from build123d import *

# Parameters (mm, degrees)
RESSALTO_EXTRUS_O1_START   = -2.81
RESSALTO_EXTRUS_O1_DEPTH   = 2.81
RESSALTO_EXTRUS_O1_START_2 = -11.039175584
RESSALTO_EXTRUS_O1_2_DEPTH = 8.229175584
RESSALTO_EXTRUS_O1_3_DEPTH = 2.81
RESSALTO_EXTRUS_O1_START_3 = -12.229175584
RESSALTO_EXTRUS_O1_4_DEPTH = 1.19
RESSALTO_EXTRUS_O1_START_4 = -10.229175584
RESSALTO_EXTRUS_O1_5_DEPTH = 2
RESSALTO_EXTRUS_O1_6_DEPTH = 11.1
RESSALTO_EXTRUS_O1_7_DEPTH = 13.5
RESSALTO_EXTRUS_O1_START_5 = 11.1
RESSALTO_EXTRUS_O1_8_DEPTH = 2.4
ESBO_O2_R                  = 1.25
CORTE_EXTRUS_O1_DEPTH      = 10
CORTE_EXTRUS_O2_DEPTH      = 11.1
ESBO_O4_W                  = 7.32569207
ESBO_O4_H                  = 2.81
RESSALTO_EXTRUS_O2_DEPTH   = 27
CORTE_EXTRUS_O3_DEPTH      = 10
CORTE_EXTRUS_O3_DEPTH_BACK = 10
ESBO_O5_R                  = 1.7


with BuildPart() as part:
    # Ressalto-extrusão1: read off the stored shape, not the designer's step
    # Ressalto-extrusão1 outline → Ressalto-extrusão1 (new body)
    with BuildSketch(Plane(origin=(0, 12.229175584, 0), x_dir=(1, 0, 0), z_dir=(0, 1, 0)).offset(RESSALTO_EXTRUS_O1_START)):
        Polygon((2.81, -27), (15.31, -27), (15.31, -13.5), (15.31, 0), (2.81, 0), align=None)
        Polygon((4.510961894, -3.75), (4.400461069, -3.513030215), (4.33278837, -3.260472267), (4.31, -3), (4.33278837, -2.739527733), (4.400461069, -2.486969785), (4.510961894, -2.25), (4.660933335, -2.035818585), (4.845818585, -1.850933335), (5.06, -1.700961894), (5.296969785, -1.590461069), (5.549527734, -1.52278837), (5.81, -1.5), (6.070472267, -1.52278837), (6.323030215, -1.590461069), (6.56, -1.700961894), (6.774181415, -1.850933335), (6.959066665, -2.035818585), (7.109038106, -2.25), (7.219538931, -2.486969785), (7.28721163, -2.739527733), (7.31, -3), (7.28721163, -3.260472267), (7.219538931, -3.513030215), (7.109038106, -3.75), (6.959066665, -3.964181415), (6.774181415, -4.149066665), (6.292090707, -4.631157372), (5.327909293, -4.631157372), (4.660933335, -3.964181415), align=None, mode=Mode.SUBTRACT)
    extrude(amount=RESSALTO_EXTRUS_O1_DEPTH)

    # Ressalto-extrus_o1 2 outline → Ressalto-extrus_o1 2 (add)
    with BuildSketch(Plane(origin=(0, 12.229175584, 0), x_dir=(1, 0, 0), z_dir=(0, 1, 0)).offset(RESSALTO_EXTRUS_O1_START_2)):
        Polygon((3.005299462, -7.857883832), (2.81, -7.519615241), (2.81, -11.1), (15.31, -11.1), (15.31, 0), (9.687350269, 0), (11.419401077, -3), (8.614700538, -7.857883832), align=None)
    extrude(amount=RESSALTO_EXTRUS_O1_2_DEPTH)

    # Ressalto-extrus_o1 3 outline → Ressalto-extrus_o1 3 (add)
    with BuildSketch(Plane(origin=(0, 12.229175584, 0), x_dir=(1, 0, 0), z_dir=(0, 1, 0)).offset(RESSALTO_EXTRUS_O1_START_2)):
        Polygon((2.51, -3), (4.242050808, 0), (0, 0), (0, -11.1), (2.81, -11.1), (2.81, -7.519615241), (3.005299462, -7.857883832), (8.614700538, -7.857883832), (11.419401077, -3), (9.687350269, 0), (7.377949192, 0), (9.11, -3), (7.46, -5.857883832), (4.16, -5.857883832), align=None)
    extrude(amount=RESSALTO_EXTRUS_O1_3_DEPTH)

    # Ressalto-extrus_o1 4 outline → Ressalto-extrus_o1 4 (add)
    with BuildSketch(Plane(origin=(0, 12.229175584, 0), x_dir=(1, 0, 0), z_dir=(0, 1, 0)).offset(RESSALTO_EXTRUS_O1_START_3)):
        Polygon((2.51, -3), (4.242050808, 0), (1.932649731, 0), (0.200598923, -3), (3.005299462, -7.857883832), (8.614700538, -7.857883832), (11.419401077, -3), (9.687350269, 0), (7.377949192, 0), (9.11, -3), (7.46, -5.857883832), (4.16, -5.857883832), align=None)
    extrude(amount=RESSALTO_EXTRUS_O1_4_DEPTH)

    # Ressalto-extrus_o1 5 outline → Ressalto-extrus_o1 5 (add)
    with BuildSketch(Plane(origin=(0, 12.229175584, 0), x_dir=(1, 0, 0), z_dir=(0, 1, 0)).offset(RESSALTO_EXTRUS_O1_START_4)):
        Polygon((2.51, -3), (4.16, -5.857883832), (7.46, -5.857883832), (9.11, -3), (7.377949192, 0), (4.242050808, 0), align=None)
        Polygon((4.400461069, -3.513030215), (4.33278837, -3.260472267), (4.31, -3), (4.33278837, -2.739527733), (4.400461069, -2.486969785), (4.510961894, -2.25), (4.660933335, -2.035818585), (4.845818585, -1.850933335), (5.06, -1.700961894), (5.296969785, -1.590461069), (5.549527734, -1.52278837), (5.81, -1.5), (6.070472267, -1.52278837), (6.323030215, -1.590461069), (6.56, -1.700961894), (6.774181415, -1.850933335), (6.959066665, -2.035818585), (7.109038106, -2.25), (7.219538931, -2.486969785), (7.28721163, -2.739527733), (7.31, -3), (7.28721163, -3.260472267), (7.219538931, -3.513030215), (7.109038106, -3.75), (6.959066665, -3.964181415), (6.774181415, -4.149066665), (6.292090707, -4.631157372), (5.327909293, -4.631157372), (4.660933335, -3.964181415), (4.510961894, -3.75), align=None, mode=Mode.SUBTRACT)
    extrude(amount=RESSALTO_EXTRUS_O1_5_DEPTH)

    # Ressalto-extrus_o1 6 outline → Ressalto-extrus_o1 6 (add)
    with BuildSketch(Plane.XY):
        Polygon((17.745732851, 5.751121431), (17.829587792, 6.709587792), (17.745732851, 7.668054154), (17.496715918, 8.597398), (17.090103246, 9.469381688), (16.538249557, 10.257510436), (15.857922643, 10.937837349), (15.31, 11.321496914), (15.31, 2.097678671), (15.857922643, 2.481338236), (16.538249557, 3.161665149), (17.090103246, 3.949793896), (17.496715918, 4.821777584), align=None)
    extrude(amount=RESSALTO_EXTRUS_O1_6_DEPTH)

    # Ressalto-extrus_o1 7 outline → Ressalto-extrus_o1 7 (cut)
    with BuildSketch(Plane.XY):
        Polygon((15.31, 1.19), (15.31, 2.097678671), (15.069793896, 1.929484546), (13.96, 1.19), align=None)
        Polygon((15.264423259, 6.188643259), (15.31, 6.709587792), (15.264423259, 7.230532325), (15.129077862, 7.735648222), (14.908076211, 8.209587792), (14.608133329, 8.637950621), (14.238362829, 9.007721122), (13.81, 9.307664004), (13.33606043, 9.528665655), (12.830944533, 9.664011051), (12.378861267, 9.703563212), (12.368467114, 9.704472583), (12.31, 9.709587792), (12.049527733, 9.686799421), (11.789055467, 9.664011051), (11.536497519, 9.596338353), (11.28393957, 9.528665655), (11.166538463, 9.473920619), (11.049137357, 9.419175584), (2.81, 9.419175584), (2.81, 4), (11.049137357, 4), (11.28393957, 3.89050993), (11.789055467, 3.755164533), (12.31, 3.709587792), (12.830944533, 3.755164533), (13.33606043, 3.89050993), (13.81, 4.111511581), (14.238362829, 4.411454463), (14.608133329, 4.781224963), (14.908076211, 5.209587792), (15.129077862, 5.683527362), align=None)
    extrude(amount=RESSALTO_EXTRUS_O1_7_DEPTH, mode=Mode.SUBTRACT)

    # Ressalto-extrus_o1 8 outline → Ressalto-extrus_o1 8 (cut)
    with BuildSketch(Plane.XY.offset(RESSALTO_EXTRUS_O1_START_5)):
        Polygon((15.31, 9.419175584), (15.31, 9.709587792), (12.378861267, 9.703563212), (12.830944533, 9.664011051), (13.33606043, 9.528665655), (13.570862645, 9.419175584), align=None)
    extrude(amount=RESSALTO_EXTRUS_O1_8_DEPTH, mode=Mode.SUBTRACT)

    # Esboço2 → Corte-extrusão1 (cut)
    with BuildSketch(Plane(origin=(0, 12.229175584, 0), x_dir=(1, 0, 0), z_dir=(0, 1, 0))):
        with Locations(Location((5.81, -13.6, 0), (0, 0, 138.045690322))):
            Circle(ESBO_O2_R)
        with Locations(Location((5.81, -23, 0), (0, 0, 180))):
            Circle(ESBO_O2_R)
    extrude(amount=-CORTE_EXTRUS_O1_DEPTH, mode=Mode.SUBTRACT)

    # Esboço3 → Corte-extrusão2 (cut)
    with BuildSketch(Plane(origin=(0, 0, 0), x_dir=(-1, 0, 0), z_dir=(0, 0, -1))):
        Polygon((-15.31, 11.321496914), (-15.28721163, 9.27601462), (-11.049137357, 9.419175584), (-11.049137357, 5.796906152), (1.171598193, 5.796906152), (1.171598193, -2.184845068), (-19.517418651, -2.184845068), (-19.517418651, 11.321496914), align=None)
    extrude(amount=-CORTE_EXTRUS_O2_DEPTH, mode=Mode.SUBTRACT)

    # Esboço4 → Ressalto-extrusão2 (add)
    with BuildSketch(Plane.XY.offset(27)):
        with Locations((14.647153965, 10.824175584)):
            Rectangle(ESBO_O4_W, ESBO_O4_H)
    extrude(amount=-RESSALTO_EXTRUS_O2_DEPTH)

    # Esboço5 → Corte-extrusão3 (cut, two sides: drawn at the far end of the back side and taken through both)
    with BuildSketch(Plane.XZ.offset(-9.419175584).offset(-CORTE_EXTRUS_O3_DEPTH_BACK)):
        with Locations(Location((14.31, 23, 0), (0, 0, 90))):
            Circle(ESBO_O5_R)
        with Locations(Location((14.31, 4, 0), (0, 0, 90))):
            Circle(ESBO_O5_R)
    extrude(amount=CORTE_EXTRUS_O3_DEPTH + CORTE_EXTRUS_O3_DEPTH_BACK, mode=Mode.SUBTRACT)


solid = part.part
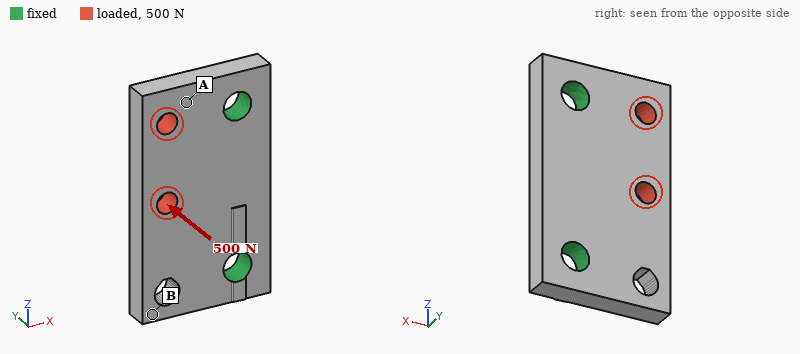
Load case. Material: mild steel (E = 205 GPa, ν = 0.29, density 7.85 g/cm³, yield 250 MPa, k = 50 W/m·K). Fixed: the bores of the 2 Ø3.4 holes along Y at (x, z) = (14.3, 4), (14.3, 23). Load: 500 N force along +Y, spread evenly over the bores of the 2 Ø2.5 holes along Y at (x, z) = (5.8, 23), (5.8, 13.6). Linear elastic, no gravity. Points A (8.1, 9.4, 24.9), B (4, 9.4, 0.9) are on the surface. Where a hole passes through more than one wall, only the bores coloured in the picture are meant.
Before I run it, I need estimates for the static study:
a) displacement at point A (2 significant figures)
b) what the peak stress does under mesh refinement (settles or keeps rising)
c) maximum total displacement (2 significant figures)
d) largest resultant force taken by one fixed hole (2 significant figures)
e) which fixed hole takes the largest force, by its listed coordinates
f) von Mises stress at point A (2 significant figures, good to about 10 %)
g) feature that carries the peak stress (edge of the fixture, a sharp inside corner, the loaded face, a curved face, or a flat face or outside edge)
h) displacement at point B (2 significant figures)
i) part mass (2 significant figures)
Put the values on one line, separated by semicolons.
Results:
7.9 µm; keeps rising; 22 µm; 380 N; (14.3, 23); 59 MPa; edge of the fixture; 5.5 µm; 8.5 g
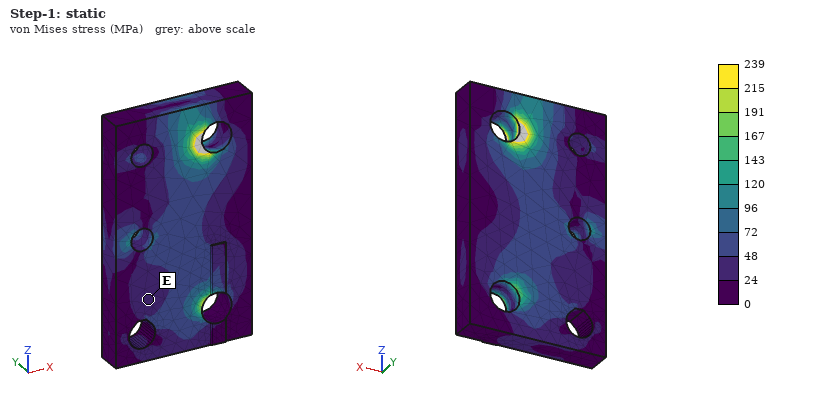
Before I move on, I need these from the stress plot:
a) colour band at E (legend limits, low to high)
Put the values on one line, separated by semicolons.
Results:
24 to 48 MPa
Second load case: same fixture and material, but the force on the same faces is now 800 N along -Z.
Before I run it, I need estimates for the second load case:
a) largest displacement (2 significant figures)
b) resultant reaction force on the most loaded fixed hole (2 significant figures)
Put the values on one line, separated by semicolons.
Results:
2.7 µm; 520 N
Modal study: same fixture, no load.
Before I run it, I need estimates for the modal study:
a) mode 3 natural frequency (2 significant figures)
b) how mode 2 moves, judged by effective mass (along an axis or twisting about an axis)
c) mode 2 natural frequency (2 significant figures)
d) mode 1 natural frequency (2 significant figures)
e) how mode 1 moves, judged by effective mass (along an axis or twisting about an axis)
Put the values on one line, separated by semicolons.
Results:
36 kHz; twisting about X; 26 kHz; 17 kHz; along Y
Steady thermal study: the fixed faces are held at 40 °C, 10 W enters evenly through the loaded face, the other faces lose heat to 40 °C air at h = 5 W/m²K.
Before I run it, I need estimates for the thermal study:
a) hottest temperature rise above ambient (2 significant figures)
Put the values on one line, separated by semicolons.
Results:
40 K
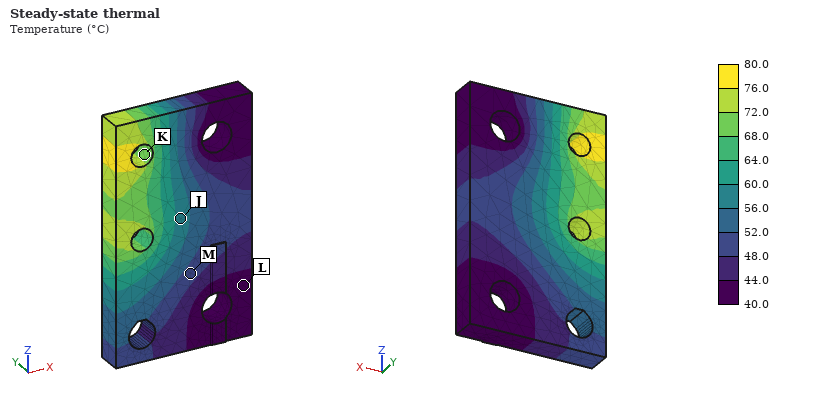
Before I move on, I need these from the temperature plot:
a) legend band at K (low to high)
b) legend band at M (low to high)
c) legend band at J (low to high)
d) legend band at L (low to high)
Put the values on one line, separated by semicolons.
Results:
68.0 to 72.0 °C; 48.0 to 52.0 °C; 56.0 to 60.0 °C; 40.0 to 44.0 °C
